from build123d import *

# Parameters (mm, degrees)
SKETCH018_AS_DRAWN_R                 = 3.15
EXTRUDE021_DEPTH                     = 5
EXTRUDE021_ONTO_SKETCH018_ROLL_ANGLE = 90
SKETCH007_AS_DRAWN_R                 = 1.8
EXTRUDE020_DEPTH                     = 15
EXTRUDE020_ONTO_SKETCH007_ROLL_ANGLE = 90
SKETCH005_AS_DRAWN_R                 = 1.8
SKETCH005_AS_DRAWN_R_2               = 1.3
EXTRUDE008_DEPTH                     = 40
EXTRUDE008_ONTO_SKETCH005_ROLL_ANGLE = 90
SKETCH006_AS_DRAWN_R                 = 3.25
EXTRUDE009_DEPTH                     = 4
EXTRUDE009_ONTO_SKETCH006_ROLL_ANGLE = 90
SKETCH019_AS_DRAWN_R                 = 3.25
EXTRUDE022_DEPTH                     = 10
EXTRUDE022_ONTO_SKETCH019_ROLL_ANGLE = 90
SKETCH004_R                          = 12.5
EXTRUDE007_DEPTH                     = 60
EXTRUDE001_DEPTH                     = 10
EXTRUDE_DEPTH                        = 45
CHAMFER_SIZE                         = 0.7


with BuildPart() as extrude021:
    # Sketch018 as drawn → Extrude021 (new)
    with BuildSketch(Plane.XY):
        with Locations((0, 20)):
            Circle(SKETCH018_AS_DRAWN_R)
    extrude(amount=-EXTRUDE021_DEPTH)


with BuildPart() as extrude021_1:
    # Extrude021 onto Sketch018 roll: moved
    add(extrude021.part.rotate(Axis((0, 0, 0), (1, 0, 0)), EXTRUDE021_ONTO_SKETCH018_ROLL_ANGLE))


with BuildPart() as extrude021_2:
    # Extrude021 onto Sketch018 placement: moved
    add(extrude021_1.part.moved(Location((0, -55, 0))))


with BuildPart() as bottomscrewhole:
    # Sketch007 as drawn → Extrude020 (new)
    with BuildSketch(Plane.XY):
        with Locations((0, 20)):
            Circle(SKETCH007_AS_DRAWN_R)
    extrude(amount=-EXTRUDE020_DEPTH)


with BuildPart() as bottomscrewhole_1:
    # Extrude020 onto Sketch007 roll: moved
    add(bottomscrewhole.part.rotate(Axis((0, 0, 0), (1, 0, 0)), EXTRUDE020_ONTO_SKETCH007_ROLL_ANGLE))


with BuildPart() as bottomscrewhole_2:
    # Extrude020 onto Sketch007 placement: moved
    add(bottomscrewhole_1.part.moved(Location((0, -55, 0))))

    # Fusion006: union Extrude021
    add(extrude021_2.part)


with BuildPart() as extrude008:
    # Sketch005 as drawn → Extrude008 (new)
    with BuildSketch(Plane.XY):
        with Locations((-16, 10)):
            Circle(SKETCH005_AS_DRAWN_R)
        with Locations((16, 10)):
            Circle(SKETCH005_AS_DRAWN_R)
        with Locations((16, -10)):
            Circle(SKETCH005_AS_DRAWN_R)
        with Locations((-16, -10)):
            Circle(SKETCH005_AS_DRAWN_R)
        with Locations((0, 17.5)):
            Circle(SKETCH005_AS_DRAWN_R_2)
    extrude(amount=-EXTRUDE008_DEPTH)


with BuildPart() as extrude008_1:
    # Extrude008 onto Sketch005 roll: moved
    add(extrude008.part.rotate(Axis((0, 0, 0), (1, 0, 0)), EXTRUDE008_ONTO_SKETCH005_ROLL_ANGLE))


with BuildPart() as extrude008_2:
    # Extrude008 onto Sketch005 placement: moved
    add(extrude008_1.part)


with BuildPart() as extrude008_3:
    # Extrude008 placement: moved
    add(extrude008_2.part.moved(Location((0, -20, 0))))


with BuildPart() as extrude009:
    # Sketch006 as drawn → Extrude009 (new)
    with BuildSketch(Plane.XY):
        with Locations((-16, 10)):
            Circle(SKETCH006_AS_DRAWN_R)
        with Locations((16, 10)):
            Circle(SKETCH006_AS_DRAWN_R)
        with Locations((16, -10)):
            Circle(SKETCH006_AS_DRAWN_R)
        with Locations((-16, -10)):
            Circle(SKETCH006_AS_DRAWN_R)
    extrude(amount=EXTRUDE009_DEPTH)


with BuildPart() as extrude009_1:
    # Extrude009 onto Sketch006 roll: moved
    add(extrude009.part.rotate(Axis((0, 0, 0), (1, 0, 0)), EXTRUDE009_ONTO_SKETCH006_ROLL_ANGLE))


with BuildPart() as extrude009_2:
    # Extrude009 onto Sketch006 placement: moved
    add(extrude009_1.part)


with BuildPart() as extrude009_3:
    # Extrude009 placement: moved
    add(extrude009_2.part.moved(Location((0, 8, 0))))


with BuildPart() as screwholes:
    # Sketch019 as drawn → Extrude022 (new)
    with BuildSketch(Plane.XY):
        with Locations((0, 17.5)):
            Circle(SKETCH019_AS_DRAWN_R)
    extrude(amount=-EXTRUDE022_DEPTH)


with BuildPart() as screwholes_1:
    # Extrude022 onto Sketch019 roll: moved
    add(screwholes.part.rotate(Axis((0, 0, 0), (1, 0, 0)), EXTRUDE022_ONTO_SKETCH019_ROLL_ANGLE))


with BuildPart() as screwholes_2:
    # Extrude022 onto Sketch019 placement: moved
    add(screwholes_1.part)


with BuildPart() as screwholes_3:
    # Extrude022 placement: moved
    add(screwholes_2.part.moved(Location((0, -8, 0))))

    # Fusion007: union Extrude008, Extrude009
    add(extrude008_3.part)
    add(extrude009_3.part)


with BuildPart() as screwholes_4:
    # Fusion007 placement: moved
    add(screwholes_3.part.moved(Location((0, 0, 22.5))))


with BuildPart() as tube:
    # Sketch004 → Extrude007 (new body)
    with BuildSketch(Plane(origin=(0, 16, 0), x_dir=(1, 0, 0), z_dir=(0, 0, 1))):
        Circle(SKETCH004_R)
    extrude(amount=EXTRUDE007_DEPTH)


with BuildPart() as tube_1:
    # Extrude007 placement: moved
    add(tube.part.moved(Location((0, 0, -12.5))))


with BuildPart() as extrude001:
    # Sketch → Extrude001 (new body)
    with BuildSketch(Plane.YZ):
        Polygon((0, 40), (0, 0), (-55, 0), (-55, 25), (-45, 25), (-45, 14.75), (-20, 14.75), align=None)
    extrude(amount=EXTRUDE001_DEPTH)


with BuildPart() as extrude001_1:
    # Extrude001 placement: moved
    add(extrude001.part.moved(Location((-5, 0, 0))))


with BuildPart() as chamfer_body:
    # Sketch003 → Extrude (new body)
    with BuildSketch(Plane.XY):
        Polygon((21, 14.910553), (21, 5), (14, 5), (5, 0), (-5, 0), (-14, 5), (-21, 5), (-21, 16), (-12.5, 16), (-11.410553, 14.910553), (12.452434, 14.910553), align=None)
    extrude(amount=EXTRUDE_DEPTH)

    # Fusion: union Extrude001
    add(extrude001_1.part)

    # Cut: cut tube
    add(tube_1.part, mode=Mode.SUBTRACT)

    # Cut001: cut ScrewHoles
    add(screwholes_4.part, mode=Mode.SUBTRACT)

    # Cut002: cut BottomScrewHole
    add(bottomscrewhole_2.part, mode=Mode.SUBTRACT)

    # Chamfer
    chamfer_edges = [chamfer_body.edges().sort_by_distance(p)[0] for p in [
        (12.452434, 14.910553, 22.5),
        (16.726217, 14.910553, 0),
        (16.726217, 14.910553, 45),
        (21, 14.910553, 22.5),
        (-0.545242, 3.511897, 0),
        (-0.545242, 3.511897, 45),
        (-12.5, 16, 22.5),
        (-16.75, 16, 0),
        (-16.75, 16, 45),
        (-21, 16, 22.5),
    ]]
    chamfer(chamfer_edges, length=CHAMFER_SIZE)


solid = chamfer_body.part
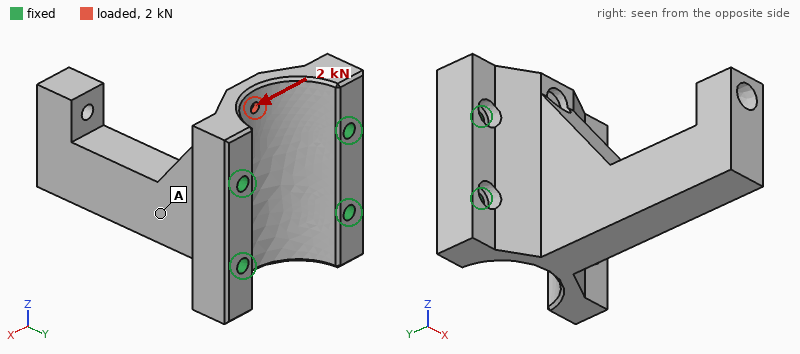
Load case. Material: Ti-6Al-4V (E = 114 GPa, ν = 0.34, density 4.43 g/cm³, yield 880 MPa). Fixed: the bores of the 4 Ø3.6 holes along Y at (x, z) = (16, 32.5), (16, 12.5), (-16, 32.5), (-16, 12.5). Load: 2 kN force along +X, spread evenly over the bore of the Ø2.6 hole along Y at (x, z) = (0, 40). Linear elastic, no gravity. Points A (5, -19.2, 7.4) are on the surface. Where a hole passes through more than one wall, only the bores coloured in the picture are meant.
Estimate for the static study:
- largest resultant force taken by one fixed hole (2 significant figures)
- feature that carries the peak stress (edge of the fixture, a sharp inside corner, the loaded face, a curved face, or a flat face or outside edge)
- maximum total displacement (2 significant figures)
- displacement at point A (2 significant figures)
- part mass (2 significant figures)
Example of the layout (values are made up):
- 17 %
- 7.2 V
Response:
- 950 N
- the loaded face
- 11 µm
- 1.8 µm
- 110 g
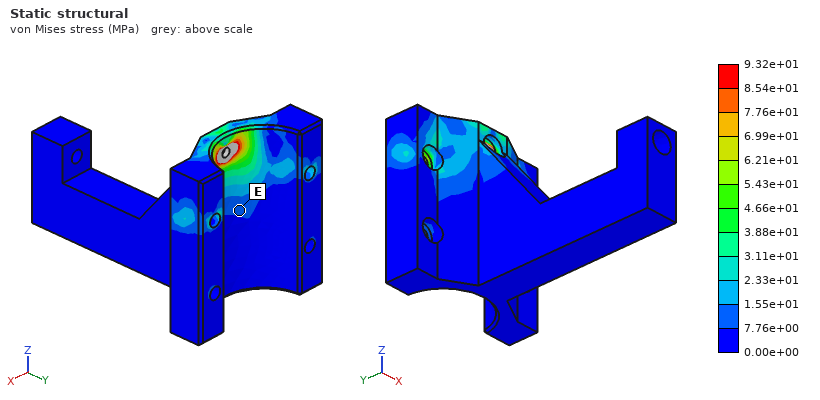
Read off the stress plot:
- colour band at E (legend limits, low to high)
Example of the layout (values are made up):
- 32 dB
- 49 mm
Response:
- 7.76e+00 to 1.55e+01 MPa
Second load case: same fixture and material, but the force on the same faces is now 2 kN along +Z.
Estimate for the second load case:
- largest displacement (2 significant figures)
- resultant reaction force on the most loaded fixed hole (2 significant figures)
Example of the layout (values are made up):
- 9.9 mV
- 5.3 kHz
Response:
- 11 µm
- 700 N
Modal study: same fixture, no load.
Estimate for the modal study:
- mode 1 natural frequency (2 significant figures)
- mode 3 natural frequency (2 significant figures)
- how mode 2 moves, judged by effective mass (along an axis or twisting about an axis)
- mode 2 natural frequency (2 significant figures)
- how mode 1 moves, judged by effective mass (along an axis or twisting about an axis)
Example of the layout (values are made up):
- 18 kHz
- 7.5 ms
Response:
- 2200 Hz
- 8800 Hz
- along Z
- 3600 Hz
- along X
